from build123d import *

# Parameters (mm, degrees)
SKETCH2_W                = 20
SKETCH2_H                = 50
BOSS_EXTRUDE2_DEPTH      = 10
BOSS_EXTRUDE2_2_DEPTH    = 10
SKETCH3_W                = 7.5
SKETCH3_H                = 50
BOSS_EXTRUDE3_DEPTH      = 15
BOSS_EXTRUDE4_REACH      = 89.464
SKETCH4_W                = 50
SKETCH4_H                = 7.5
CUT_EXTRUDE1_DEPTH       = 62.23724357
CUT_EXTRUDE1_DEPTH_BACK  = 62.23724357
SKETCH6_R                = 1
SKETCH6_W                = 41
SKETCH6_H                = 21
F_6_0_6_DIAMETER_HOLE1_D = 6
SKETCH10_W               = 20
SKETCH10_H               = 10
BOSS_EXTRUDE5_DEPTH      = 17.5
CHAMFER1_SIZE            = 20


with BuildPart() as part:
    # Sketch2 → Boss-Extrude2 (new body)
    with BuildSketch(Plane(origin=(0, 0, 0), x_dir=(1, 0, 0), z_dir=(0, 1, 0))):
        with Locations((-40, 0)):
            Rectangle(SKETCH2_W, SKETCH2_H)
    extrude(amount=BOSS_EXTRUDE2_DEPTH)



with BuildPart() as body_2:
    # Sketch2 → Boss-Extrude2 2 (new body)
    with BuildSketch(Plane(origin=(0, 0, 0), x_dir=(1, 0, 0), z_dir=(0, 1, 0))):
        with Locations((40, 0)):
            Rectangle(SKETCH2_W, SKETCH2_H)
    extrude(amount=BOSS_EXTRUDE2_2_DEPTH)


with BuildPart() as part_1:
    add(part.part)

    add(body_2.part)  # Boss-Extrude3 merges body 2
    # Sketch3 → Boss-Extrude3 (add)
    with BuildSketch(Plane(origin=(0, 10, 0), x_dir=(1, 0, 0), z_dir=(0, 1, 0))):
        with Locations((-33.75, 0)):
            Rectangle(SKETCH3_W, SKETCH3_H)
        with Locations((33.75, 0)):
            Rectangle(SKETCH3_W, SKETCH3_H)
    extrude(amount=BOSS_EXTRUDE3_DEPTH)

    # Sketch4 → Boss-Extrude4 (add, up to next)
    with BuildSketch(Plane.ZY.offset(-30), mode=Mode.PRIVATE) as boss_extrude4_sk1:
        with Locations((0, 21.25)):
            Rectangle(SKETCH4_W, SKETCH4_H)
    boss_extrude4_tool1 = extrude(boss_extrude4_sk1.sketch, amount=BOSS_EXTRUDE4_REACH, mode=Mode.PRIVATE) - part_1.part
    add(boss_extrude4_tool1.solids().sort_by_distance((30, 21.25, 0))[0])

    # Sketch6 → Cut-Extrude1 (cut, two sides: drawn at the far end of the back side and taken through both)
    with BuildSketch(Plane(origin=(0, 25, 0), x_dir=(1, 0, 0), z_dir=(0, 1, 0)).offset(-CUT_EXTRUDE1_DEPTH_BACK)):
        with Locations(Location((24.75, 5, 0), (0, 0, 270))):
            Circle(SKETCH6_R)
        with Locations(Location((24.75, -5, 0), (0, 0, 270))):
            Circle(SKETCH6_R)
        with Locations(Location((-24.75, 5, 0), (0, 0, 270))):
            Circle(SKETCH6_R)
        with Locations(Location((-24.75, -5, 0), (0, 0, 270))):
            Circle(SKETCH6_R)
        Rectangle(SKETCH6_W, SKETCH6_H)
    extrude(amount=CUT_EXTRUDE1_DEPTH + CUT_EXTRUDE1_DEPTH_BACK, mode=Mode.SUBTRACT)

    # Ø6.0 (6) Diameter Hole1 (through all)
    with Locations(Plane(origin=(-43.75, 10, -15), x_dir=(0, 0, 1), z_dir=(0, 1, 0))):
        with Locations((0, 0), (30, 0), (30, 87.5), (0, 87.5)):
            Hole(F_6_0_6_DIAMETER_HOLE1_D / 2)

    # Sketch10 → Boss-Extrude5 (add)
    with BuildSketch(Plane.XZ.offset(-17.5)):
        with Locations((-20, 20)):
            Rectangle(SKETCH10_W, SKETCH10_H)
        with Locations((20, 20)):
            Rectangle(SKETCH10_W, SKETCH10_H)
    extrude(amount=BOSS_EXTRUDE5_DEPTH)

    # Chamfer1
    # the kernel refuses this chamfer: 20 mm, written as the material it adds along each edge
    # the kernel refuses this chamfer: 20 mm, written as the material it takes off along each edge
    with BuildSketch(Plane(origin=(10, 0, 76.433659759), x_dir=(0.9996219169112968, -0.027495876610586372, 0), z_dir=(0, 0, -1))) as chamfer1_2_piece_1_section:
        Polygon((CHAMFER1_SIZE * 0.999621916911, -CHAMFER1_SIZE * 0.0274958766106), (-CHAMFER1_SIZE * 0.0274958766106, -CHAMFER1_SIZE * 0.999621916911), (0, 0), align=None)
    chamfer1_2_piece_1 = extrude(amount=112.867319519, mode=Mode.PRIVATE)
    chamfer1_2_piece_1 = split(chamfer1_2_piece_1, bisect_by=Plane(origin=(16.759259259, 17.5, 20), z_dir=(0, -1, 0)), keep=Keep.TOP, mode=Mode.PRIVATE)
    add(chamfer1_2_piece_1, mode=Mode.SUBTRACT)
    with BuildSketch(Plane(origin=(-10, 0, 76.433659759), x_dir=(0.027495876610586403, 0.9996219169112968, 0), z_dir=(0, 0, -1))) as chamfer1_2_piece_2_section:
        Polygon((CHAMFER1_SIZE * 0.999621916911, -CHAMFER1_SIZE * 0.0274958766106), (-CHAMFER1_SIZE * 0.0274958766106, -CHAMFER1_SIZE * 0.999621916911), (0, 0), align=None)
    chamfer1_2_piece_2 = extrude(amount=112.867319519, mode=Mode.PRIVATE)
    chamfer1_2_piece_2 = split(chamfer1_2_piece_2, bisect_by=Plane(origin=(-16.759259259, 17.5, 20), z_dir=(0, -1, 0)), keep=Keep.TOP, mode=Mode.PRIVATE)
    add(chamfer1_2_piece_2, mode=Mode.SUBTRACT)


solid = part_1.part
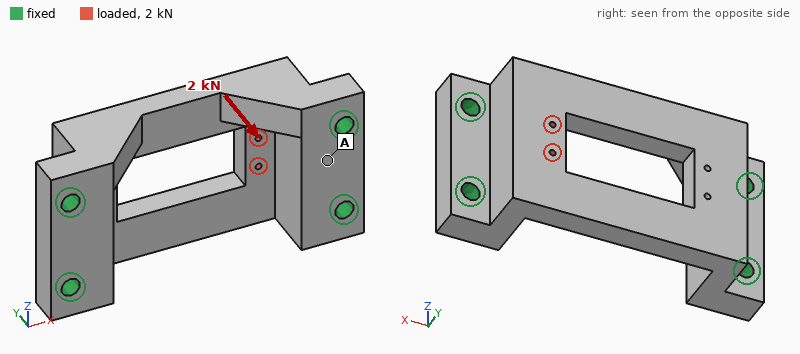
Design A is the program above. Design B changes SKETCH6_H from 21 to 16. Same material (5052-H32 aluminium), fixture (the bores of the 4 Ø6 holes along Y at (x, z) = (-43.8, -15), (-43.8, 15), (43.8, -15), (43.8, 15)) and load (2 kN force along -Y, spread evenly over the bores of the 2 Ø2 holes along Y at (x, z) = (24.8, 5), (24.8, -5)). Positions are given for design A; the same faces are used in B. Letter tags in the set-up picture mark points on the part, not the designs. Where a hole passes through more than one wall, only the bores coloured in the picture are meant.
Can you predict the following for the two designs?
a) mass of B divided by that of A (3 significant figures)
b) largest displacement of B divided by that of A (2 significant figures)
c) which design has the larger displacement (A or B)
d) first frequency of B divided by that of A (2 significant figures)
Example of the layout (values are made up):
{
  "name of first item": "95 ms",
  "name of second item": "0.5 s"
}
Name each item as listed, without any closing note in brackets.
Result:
{
  "mass of B divided by that of A": "1.03",
  "largest displacement of B divided by that of A": "0.89",
  "which design has the larger displacement": "A",
  "first frequency of B divided by that of A": "0.99"
}
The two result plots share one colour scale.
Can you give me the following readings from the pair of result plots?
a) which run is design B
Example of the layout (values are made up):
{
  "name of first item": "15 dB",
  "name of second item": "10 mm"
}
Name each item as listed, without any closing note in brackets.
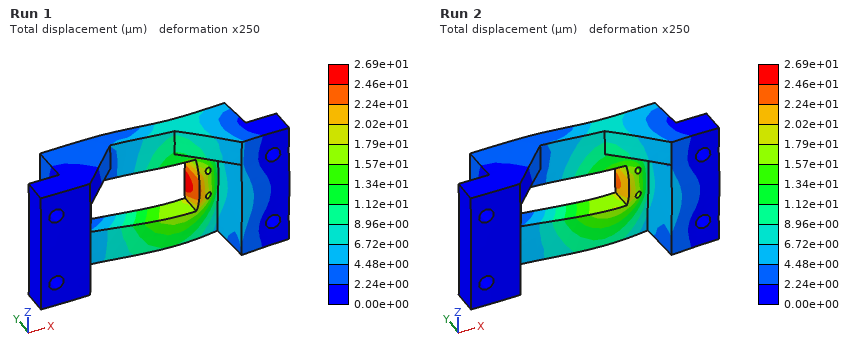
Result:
{
  "which run is design B": "Run 2"
}
